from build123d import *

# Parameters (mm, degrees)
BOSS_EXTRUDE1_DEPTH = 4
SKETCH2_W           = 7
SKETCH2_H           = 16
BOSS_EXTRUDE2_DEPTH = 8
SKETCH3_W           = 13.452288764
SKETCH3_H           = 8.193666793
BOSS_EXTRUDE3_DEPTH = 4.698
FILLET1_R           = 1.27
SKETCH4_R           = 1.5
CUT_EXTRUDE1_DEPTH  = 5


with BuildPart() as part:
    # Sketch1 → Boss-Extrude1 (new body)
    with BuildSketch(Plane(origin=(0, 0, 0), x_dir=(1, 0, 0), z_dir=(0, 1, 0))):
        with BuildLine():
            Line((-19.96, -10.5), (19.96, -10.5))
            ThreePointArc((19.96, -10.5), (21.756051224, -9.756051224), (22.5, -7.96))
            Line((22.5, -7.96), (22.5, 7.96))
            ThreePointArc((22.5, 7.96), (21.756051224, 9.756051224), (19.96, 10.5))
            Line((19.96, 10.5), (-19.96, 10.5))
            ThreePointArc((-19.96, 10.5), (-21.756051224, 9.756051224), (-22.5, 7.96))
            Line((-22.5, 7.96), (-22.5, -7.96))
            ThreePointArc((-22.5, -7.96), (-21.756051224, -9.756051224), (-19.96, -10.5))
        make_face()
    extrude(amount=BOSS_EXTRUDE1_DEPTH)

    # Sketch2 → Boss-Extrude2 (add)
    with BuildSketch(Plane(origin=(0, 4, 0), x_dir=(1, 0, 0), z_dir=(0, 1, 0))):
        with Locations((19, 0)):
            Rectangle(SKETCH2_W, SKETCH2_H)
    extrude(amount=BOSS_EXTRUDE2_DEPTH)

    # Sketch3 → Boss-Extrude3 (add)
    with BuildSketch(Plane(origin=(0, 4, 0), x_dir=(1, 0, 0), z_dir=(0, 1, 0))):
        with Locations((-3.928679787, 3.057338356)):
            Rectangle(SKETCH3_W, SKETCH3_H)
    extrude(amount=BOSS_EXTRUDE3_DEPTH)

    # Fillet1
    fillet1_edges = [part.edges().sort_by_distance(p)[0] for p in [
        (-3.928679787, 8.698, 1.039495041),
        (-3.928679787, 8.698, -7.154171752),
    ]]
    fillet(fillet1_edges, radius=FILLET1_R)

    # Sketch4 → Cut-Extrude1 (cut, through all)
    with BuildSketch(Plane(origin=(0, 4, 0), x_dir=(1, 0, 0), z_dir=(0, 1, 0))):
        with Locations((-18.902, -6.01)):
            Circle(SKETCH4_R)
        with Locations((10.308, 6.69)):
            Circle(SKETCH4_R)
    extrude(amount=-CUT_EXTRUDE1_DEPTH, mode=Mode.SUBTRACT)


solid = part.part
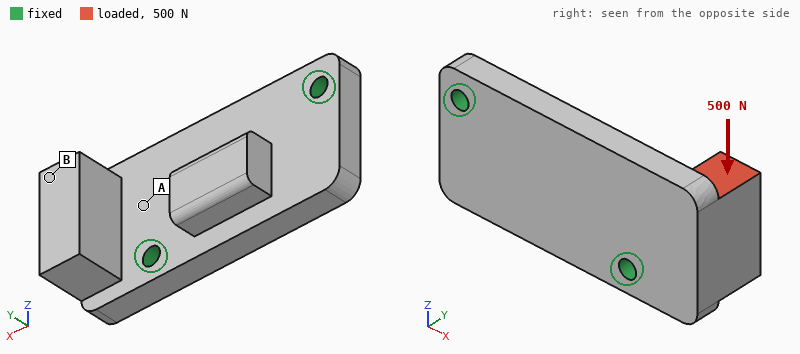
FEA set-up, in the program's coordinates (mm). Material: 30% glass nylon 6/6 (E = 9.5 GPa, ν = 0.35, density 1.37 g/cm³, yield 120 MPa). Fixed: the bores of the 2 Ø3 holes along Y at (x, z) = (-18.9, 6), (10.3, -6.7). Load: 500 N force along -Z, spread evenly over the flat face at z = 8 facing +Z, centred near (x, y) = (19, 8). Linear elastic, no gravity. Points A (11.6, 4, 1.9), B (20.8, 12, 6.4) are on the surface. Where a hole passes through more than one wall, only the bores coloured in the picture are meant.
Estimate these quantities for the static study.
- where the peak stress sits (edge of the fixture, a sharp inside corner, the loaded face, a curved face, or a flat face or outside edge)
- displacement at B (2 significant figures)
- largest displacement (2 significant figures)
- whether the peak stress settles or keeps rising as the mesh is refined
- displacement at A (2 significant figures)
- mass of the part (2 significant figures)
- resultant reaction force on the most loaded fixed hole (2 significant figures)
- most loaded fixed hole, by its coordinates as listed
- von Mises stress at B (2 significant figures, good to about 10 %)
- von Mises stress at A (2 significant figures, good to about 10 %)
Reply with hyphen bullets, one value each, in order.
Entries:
- edge of the fixture
- 0.32 mm
- 0.35 mm
- keeps rising
- 0.11 mm
- 7.0 g
- 580 N
- (10.3, -6.7)
- 9.2 MPa
- 26 MPa
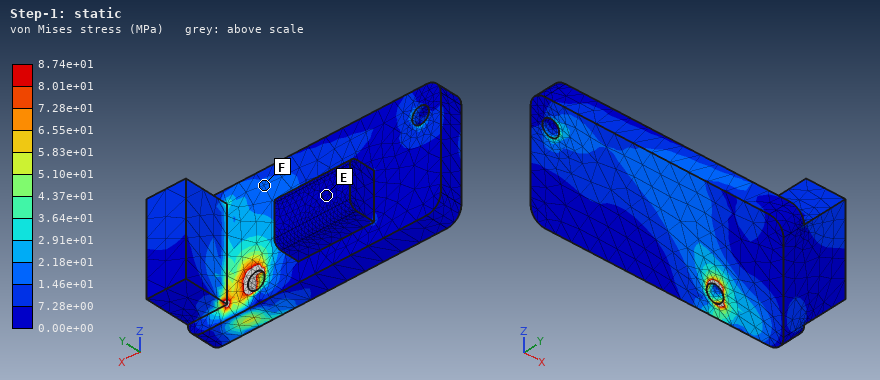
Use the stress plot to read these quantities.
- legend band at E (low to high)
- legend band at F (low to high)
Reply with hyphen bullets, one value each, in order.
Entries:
- 0.00e+00 to 7.28e+00 MPa
- 1.46e+01 to 2.18e+01 MPa
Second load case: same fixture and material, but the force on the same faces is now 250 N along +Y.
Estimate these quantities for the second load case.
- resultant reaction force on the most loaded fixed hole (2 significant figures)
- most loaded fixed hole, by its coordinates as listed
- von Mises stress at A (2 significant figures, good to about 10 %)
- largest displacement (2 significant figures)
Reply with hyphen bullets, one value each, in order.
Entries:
- 270 N
- (10.3, -6.7)
- 27 MPa
- 0.52 mm
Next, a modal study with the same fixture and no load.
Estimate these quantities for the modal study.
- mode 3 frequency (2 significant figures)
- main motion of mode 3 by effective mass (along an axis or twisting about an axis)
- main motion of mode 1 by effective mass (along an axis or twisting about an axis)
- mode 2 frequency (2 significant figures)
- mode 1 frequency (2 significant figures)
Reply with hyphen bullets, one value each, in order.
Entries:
- 6800 Hz
- along Y
- along Y
- 5700 Hz
- 3600 Hz
